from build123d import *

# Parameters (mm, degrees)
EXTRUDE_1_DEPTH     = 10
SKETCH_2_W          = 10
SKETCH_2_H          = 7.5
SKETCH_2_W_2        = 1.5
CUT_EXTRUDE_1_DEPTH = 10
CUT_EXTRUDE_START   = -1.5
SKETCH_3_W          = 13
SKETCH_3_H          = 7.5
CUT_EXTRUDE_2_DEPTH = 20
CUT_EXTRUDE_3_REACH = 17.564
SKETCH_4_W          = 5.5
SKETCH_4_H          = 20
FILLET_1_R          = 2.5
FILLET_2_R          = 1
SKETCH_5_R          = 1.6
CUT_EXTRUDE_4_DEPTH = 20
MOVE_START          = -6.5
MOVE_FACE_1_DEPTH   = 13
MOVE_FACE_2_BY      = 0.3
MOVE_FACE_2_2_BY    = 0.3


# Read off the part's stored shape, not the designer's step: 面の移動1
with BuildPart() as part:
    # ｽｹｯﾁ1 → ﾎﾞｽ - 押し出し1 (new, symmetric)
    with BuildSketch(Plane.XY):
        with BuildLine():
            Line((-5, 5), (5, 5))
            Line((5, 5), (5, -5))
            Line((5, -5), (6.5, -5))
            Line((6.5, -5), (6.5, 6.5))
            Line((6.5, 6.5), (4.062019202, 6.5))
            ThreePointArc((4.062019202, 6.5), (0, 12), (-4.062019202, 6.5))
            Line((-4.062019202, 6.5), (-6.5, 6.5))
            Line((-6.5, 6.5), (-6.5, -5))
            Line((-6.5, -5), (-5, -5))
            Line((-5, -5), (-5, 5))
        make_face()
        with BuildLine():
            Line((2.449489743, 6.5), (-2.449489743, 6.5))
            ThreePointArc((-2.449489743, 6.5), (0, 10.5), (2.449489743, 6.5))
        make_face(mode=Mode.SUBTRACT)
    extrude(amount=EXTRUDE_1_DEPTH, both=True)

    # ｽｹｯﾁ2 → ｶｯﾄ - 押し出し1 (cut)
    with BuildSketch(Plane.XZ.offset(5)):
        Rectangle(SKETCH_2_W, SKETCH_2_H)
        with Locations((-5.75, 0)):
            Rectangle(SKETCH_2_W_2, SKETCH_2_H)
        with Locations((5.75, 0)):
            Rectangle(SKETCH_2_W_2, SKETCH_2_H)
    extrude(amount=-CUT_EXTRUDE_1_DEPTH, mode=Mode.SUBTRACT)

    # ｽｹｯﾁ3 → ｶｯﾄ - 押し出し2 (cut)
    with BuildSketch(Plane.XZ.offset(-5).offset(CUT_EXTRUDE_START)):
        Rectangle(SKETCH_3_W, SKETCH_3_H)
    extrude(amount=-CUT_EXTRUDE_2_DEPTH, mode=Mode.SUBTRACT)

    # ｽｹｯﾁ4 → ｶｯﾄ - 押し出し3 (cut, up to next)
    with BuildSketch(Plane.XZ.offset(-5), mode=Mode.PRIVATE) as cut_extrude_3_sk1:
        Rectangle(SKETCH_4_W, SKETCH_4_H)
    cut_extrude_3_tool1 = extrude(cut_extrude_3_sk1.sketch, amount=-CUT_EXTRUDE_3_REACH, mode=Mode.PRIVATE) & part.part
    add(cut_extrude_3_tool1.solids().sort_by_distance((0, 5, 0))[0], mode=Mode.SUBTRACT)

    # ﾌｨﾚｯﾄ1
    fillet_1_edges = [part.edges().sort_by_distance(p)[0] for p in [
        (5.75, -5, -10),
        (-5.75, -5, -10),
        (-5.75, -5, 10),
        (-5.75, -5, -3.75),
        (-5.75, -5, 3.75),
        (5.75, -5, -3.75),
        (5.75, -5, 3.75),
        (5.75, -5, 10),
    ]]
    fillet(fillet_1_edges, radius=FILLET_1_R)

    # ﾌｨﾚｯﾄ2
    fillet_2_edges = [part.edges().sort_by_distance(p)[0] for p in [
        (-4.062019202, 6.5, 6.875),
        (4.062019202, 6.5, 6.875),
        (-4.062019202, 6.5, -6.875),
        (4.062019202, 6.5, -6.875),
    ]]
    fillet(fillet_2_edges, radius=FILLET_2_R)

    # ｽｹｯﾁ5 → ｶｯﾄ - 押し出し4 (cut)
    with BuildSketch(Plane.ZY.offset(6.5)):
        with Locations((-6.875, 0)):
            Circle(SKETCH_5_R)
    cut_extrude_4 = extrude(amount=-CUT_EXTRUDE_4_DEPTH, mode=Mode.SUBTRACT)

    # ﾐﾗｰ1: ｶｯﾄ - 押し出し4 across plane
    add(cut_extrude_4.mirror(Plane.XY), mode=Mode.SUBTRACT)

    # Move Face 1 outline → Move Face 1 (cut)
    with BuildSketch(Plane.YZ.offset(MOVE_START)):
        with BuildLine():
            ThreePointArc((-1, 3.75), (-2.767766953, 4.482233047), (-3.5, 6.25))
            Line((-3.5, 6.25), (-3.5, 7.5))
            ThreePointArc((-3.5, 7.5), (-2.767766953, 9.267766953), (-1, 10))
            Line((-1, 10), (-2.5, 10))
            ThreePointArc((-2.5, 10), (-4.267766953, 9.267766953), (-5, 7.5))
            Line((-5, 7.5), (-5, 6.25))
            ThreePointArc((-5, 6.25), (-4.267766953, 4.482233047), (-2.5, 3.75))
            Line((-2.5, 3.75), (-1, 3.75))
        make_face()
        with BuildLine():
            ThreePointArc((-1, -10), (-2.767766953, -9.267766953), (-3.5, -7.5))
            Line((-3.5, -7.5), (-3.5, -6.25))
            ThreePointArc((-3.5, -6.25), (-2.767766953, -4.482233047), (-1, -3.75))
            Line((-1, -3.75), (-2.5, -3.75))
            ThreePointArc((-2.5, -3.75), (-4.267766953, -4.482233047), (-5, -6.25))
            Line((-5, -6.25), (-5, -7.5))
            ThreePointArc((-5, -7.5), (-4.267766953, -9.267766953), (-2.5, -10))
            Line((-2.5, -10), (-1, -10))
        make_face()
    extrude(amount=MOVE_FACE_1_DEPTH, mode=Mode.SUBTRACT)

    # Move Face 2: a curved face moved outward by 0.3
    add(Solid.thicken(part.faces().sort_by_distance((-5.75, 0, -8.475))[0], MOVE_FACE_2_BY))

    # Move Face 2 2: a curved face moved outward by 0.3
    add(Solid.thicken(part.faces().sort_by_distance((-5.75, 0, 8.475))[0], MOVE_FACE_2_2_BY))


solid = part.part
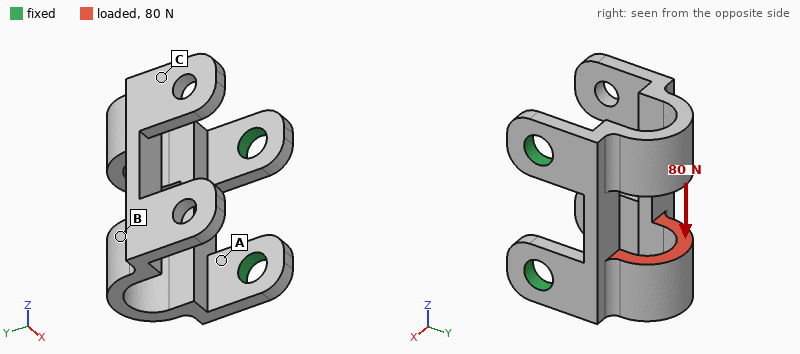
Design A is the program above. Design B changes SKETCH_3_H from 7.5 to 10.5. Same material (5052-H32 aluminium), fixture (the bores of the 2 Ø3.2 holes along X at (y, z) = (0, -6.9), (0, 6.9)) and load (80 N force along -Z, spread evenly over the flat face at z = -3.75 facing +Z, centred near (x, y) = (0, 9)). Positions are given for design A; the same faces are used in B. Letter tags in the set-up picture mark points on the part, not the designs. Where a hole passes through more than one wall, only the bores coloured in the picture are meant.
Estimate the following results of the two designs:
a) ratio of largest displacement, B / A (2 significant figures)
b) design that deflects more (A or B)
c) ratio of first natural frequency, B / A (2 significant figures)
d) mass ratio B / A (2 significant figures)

1.2
B
0.93
0.92
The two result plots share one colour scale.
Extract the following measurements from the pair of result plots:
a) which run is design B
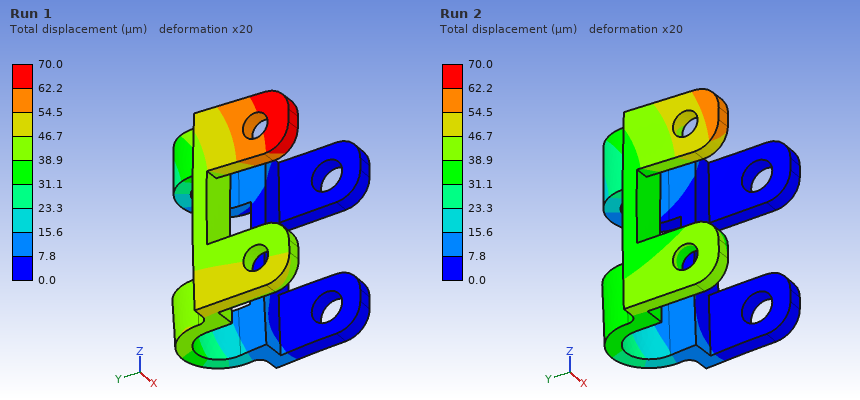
Run 1
